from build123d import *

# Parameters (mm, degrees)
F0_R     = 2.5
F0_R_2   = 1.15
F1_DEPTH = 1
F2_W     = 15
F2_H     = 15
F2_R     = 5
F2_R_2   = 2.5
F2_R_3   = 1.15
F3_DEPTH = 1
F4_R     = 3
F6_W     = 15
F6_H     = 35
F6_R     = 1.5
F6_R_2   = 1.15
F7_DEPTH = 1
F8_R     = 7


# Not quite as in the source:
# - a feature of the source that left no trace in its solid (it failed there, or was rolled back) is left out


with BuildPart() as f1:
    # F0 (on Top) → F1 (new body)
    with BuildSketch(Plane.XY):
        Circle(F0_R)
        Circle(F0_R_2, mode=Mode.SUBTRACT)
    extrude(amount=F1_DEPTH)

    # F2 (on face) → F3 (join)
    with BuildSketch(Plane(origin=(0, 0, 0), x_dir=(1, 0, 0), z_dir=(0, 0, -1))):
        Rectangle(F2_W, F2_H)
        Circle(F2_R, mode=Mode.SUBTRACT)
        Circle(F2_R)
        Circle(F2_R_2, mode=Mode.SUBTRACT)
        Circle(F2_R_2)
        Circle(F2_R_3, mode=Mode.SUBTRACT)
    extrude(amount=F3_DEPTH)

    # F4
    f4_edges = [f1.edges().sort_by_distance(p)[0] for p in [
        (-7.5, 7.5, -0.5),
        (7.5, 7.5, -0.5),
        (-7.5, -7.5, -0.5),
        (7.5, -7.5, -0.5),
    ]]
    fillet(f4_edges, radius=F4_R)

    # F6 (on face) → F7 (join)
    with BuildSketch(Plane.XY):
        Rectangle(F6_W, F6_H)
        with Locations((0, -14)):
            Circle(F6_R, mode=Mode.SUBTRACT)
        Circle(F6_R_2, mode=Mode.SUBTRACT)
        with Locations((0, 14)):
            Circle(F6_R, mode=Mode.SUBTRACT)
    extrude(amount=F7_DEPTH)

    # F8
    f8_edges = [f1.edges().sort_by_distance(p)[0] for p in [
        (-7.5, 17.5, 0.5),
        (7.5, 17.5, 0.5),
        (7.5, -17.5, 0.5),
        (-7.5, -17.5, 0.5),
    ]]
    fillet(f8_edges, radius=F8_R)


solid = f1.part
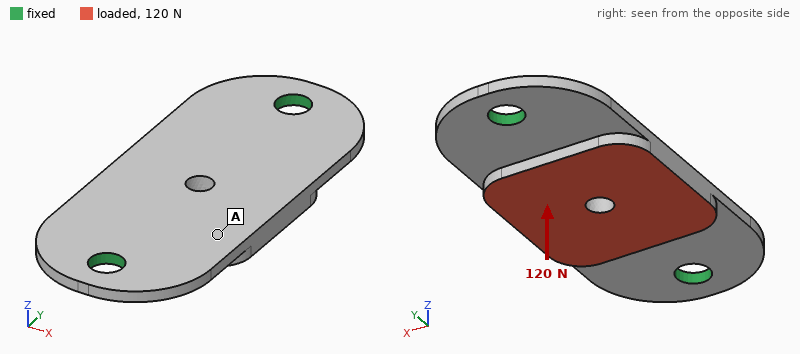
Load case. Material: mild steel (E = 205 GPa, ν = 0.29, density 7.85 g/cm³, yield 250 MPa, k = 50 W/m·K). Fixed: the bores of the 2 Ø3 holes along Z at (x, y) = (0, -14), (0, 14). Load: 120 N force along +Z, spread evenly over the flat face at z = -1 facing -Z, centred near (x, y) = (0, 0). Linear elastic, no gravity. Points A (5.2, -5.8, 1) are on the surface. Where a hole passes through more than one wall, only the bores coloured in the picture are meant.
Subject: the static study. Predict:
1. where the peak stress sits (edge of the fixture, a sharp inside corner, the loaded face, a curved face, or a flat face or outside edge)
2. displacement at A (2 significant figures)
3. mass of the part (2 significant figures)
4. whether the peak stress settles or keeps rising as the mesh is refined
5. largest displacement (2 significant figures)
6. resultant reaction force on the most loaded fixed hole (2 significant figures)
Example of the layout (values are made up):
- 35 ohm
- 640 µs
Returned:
- edge of the fixture
- 12 µm
- 5.3 g
- keeps rising
- 15 µm
- 120 N
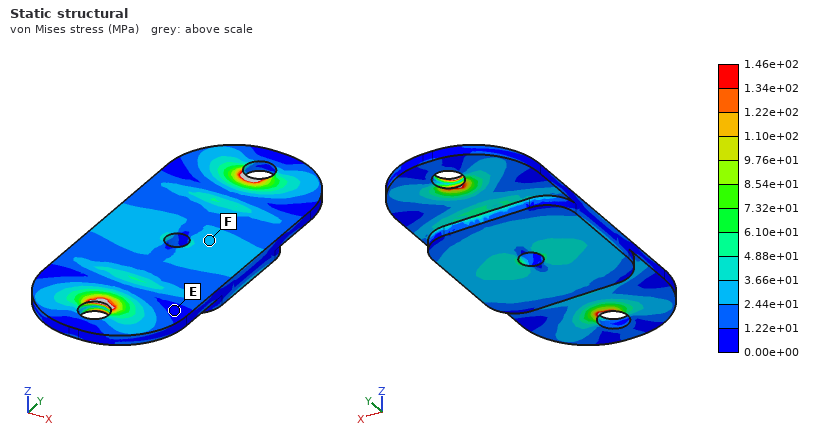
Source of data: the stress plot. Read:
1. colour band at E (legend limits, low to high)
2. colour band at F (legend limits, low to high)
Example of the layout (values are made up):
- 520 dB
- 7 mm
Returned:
- 0.00e+00 to 1.22e+01 MPa
- 2.44e+01 to 3.66e+01 MPa
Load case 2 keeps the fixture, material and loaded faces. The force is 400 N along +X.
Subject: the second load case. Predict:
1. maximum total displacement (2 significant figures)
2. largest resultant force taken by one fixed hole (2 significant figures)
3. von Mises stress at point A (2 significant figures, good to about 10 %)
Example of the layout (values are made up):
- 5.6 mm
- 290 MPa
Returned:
- 32 µm
- 200 N
- 45 MPa
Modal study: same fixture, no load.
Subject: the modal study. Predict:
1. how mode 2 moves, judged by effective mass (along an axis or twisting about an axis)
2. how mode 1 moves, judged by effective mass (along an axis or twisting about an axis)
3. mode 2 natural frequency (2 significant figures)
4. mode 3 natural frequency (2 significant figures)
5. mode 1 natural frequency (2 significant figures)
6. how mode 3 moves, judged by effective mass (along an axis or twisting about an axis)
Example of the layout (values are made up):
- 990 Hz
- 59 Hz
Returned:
- along Z
- twisting about Y
- 8100 Hz
- 19 kHz
- 7200 Hz
- twisting about X
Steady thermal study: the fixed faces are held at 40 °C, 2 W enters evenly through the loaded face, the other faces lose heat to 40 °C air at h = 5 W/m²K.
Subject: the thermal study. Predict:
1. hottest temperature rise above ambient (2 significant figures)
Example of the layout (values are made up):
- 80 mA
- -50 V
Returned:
- 13 K
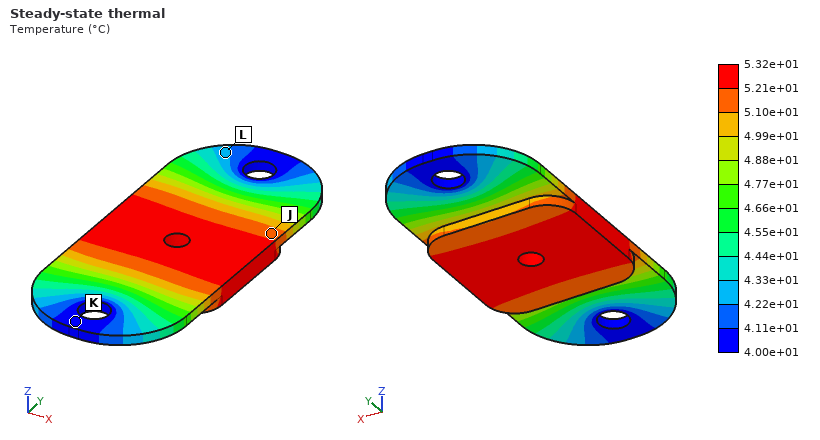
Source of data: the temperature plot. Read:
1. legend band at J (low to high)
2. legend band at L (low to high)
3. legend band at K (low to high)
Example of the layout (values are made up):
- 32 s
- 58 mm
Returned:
- 5.10e+01 to 5.21e+01 °C
- 4.22e+01 to 4.33e+01 °C
- 4.00e+01 to 4.11e+01 °C
